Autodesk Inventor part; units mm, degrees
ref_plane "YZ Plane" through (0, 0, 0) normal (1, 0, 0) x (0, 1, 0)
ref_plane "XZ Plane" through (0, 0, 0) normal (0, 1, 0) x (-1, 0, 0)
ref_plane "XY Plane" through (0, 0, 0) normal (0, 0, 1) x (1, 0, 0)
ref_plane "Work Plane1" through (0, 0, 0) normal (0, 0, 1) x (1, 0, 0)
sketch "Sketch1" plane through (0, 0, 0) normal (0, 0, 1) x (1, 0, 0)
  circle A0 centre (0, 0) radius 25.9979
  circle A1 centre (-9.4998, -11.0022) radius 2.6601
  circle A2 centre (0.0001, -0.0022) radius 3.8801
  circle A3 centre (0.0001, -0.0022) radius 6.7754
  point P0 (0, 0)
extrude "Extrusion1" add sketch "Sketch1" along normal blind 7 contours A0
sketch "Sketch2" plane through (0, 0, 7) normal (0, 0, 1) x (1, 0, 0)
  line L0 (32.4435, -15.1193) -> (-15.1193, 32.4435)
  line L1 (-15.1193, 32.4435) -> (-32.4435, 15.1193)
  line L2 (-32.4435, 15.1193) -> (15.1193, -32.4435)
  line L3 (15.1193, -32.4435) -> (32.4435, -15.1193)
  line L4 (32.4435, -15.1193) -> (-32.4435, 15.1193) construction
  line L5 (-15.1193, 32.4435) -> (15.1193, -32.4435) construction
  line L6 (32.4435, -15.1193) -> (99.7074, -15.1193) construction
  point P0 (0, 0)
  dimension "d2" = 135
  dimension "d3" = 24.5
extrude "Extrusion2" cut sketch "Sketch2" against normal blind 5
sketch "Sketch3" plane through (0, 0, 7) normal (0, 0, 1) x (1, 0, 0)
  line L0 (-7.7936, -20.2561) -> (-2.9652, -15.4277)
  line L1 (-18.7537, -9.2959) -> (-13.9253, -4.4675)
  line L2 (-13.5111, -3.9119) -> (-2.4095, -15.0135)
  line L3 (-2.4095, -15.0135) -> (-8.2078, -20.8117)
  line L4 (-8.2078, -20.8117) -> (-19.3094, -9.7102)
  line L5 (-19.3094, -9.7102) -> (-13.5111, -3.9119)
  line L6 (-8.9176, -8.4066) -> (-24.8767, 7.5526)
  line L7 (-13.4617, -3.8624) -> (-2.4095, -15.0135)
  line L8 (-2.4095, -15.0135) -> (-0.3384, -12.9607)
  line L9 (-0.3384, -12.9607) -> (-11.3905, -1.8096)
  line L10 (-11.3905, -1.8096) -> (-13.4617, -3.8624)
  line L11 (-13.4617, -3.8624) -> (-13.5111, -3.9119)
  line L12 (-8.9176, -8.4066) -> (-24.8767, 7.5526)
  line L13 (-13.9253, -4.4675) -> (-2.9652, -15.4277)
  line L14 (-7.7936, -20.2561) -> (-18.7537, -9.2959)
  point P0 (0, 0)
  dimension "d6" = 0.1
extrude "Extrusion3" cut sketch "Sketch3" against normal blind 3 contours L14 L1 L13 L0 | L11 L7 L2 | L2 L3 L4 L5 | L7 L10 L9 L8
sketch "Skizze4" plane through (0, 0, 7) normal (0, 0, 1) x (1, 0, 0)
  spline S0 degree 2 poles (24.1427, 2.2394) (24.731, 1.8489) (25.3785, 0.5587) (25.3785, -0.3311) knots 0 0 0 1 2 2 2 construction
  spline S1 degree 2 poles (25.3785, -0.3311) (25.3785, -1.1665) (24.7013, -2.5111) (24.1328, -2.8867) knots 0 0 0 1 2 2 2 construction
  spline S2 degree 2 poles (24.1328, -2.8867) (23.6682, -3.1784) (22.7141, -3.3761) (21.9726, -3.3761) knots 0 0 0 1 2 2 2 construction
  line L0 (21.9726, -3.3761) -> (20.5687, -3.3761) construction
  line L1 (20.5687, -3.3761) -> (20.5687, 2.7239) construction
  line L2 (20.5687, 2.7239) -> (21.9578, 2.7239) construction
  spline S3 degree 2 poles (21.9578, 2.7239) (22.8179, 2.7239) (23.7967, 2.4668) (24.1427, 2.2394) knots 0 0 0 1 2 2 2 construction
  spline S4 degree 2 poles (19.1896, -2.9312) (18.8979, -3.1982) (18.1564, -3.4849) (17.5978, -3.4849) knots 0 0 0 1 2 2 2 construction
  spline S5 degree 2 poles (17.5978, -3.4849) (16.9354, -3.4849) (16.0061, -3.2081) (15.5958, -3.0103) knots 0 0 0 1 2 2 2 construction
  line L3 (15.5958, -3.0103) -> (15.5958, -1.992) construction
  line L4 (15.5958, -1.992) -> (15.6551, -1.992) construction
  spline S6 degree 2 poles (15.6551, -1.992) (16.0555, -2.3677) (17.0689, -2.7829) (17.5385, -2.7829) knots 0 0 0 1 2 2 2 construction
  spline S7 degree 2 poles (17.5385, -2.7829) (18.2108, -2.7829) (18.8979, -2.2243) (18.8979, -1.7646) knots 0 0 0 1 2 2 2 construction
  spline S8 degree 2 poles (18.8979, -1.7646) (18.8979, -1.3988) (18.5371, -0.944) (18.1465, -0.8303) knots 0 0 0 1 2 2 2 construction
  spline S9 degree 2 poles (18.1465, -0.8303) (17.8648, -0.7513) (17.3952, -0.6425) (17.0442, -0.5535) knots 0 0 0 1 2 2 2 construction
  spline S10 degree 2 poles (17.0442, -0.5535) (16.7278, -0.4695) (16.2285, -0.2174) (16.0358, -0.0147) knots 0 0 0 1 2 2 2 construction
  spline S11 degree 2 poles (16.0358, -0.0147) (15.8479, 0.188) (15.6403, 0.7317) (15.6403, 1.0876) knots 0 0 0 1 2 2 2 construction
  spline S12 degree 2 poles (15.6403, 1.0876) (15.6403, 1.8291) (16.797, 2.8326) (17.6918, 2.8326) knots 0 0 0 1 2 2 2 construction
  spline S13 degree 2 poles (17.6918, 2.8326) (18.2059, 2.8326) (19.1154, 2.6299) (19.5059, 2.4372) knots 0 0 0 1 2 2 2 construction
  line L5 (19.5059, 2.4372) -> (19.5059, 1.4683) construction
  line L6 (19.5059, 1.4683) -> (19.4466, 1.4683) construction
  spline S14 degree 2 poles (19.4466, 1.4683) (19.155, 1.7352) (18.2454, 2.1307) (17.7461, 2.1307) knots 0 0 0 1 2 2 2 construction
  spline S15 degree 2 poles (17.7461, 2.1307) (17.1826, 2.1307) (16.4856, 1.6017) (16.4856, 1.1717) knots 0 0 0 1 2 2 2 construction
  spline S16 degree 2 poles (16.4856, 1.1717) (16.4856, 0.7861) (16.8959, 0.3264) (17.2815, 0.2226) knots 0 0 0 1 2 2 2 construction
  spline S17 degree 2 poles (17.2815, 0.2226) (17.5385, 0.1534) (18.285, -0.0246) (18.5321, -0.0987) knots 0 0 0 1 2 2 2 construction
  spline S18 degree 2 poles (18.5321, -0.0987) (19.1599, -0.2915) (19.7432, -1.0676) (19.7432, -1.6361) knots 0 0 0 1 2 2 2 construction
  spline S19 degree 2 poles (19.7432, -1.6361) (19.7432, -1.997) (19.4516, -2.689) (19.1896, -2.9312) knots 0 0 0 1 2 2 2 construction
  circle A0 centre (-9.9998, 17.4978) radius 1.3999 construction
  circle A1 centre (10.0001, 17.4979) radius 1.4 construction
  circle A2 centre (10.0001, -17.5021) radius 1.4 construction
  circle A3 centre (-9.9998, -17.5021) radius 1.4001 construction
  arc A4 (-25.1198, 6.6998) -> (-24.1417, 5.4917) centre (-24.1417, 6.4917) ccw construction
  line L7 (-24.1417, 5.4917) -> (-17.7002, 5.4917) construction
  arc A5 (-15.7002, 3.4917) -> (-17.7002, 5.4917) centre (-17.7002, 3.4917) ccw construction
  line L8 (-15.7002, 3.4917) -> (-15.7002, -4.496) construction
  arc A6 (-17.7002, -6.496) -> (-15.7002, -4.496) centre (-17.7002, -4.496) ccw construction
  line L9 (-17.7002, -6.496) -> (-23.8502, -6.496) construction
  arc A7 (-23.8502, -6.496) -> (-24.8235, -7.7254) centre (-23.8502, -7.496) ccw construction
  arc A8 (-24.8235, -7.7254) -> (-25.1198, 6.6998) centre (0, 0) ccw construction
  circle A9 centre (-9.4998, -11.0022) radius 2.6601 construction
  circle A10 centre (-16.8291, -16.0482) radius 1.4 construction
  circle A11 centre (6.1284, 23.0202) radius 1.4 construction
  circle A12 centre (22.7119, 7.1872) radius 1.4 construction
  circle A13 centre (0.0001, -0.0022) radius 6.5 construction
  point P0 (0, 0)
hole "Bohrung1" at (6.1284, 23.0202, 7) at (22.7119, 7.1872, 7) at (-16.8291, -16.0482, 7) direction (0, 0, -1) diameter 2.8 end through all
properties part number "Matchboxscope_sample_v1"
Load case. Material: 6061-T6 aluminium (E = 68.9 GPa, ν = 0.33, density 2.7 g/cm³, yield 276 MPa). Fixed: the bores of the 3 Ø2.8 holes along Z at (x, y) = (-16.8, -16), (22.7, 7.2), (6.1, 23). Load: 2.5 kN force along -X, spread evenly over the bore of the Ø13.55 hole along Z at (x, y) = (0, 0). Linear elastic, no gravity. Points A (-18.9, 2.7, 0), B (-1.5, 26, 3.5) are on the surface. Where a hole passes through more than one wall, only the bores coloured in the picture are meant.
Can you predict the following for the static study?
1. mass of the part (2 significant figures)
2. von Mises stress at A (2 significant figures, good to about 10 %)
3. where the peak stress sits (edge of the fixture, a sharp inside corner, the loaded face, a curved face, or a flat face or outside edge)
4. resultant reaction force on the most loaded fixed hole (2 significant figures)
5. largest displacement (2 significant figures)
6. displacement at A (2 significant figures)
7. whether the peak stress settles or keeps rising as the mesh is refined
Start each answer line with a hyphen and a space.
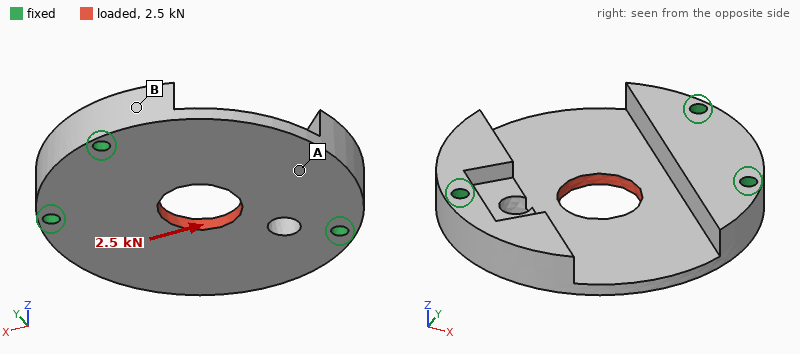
- 21 g
- 17 MPa
- edge of the fixture
- 1.0 kN
- 18 µm
- 12 µm
- keeps rising
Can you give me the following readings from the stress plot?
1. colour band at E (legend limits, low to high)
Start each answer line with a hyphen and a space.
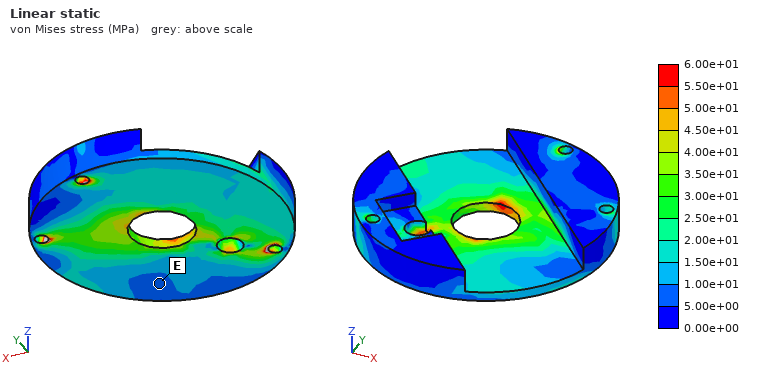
- 5.00e+00 to 1.00e+01 MPa
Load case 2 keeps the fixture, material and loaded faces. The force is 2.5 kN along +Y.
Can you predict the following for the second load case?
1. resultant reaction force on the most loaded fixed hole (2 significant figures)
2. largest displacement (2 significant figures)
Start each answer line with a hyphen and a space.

- 1.0 kN
- 19 µm
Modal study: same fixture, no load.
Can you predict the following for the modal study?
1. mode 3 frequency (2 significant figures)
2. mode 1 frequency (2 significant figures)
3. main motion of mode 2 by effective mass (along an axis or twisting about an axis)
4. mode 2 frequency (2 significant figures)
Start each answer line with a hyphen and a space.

- 14 kHz
- 7300 Hz
- along Z
- 8100 Hz
